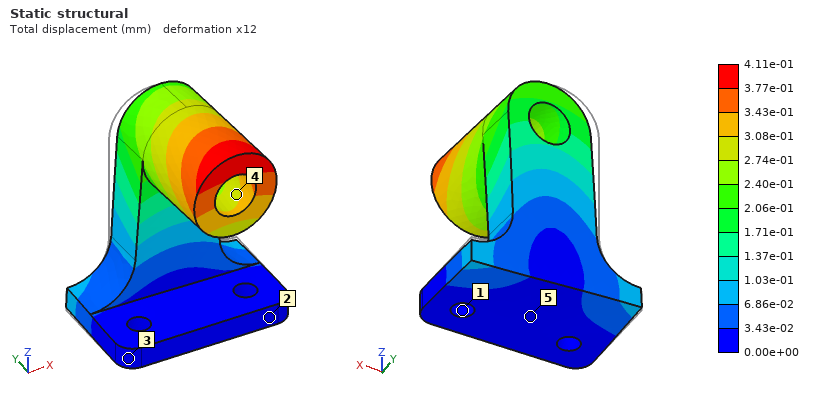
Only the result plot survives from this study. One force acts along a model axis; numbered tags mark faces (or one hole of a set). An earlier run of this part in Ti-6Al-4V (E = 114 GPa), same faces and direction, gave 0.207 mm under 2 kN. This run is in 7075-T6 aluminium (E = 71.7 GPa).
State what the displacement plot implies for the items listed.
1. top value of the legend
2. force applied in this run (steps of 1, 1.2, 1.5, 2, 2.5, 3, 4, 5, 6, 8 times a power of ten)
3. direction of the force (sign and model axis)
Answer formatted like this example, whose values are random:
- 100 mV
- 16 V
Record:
- 4.11e-01 mm
- 2.5 kN
- +X
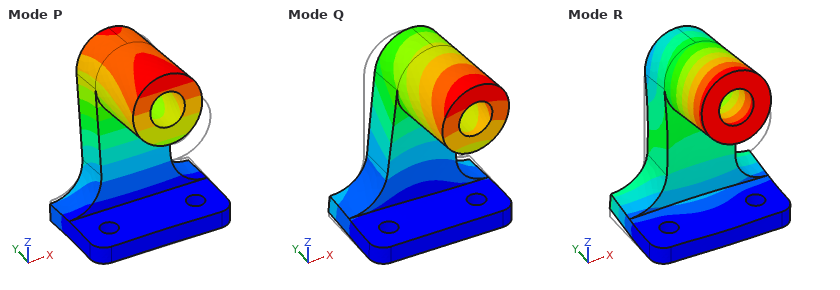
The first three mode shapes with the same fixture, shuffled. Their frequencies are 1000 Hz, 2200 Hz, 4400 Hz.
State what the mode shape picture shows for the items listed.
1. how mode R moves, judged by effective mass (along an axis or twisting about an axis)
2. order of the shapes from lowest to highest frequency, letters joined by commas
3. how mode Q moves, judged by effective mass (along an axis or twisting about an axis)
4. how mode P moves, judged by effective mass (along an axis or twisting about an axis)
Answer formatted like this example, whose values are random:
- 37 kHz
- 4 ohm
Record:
- along Z
- P, Q, R
- along X
- along Y
